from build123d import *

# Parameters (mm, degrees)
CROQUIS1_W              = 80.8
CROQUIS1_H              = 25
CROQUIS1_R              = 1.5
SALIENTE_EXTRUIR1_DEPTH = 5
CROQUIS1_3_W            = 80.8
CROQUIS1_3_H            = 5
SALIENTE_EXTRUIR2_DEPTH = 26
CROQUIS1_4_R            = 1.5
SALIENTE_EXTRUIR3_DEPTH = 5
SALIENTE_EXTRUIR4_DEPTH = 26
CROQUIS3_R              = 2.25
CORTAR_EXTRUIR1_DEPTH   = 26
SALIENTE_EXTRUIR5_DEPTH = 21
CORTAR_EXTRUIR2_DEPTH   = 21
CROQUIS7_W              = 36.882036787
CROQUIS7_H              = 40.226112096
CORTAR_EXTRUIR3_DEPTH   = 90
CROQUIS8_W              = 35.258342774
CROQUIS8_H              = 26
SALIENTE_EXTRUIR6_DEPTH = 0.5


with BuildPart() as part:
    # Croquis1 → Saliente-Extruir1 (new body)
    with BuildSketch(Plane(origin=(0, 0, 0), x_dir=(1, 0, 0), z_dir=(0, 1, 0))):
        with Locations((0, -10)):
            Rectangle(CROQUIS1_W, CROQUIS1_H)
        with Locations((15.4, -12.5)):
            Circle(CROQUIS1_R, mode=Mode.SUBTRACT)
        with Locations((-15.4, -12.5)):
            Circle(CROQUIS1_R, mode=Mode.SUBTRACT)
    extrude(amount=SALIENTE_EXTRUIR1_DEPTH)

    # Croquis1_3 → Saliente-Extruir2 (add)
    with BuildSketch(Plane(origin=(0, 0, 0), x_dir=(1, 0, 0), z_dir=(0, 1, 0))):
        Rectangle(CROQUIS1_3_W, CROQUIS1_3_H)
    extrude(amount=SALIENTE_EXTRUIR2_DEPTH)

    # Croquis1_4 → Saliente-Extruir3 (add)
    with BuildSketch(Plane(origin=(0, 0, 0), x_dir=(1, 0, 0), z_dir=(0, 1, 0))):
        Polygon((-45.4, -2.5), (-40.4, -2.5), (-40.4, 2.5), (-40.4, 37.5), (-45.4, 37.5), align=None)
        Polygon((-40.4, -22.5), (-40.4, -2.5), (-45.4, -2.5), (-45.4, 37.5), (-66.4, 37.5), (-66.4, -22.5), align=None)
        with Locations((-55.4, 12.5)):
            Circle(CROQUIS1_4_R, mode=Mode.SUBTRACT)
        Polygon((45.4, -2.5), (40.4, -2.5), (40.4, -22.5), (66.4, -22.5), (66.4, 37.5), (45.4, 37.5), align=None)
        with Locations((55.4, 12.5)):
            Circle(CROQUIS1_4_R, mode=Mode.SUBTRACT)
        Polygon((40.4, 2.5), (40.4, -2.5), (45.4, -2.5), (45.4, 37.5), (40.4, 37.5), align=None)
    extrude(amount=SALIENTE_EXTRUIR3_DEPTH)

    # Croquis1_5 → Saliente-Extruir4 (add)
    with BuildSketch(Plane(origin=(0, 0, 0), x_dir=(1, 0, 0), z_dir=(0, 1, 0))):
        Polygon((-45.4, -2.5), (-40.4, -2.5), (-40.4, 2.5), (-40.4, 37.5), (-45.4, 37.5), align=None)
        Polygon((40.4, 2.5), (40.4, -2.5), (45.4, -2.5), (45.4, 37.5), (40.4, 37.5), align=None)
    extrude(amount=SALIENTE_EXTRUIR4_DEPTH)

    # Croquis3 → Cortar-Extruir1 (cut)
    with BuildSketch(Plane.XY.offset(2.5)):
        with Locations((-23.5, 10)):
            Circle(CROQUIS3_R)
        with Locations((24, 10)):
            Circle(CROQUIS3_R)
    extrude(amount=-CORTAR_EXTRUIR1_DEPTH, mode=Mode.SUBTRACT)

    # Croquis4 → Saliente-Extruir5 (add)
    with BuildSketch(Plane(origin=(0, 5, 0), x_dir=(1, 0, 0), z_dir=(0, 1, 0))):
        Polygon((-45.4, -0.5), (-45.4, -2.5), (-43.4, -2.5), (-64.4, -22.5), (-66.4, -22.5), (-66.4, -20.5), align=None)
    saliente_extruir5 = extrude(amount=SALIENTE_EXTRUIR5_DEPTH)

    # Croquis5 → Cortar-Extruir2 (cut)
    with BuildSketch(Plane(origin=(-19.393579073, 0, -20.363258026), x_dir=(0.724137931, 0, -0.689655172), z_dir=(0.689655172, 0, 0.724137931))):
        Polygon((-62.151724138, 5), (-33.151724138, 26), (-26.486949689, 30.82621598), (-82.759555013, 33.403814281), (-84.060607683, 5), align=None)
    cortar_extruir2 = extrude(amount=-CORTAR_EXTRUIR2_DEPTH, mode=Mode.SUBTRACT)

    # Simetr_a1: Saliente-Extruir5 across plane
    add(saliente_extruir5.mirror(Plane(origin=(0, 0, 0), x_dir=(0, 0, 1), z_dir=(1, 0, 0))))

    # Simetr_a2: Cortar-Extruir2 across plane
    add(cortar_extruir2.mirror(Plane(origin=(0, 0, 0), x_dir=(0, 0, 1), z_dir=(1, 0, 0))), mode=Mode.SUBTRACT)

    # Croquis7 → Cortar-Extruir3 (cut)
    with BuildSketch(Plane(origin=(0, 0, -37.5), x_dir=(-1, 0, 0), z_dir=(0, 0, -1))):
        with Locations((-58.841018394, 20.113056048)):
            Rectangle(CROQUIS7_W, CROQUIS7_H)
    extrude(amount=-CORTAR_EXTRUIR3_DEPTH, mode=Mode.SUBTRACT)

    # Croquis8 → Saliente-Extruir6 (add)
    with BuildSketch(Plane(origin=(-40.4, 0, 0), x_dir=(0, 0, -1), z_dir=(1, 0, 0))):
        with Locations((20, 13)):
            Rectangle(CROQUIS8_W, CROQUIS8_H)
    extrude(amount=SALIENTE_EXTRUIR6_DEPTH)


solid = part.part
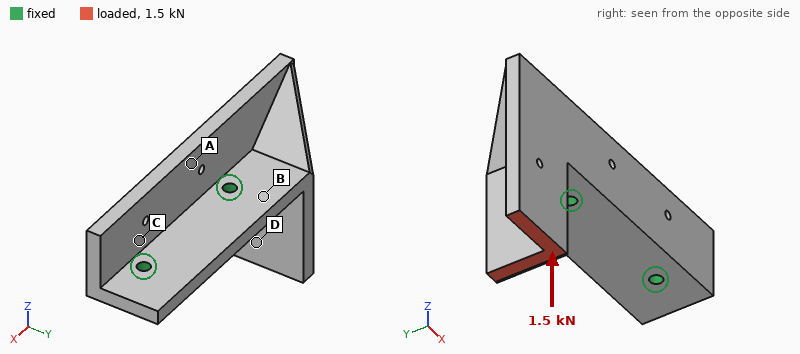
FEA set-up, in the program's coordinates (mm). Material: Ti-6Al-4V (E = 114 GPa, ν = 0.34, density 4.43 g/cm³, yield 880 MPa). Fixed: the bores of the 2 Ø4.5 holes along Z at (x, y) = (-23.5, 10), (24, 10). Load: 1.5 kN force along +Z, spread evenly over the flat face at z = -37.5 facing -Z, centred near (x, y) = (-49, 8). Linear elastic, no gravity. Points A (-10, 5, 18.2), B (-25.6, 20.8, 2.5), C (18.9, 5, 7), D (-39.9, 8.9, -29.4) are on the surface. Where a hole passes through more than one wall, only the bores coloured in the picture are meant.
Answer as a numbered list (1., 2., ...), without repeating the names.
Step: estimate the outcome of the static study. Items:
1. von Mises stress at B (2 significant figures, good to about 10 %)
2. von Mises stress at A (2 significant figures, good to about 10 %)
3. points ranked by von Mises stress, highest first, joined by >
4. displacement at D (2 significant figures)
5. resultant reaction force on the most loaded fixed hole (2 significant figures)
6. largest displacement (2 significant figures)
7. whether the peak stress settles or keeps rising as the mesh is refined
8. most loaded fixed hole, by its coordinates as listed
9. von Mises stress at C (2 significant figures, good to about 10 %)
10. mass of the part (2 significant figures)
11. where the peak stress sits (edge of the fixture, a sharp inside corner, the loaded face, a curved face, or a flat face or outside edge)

1. 40 MPa
2. 25 MPa
3. B > A > C > D
4. 55 µm
5. 2.3 kN
6. 88 µm
7. keeps rising
8. (-23.5, 10)
9. 17 MPa
10. 140 g
11. edge of the fixture
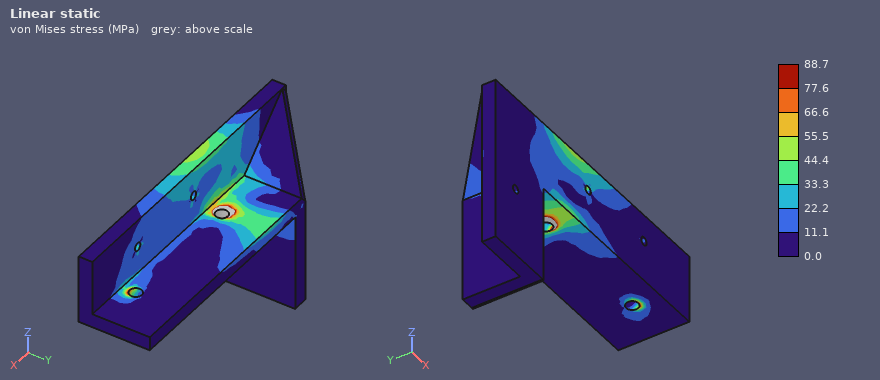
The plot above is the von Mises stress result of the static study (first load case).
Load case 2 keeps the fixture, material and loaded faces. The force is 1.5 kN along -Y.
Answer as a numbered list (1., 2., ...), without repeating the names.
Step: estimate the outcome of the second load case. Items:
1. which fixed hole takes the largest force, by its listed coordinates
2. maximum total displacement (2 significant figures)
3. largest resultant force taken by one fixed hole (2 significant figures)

1. (-23.5, 10)
2. 0.61 mm
3. 2.2 kN
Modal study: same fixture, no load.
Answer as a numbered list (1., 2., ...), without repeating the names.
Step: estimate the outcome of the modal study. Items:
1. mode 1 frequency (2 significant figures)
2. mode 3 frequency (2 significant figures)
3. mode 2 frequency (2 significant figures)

1. 2000 Hz
2. 4100 Hz
3. 2800 Hz
